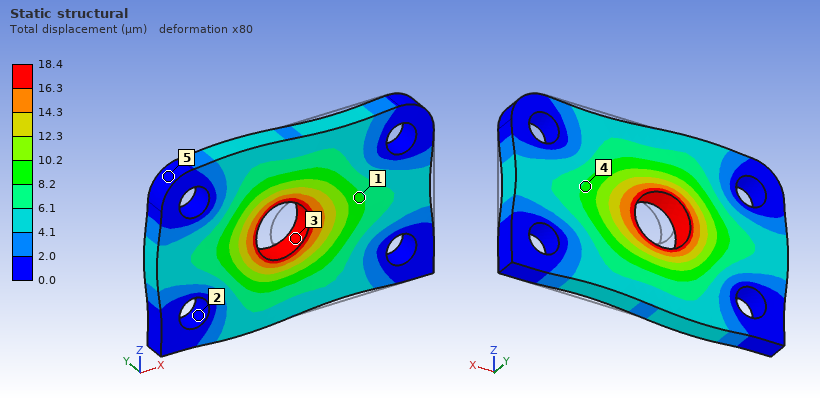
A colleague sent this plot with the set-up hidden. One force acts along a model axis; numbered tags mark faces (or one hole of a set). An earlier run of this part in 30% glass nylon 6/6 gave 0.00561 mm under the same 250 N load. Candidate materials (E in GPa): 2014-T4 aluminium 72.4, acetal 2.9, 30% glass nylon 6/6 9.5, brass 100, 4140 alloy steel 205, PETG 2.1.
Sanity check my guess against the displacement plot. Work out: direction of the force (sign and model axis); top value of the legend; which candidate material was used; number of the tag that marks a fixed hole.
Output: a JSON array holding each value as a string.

["-X", "18.4 µm", "acetal", "2"]
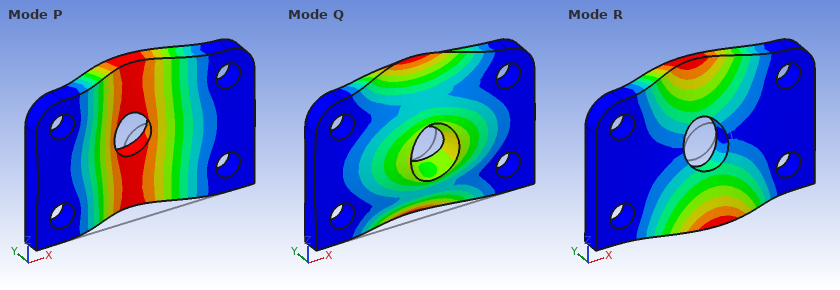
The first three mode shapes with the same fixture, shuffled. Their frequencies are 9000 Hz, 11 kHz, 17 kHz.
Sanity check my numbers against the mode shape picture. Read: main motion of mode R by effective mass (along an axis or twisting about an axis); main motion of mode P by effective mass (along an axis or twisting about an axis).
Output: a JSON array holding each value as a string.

["twisting about X", "along Y"]
